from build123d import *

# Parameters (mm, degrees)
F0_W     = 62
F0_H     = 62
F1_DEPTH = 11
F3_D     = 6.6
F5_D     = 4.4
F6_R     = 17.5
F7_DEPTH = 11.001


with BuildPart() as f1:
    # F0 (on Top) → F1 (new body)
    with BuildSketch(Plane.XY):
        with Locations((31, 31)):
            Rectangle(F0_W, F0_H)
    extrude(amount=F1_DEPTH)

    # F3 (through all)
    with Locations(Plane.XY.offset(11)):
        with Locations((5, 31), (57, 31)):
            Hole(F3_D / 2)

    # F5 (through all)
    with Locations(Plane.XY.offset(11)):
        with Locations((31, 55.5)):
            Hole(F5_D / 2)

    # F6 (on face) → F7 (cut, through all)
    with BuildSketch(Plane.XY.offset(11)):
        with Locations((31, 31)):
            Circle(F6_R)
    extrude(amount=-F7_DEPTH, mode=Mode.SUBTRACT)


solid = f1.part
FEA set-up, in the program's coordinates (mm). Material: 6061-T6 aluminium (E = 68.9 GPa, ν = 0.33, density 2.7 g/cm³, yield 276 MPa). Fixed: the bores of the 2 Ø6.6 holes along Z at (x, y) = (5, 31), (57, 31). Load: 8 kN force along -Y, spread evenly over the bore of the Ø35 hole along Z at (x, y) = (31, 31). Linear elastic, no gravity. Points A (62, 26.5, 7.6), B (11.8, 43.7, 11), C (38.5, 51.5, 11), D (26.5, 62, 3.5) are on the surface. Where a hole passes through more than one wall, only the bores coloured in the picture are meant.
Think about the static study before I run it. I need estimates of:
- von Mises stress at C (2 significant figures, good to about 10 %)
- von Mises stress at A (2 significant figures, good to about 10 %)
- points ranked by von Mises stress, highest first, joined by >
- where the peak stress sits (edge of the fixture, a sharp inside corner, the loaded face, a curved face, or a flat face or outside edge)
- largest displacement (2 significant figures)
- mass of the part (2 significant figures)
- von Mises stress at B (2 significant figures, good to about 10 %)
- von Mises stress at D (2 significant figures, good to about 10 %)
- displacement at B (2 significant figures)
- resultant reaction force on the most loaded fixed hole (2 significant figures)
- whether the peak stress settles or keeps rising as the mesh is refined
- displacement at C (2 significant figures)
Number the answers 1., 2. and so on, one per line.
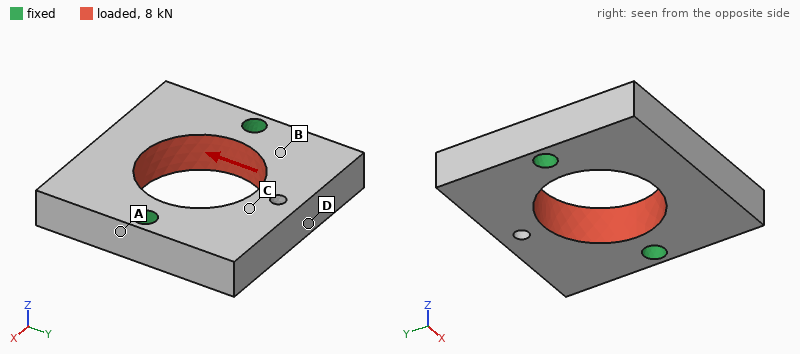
1. 8.7 MPa
2. 3.5 MPa
3. D > B > C > A
4. edge of the fixture
5. 9.3 µm
6. 83 g
7. 12 MPa
8. 18 MPa
9. 3.1 µm
10. 4.0 kN
11. keeps rising
12. 7.4 µm
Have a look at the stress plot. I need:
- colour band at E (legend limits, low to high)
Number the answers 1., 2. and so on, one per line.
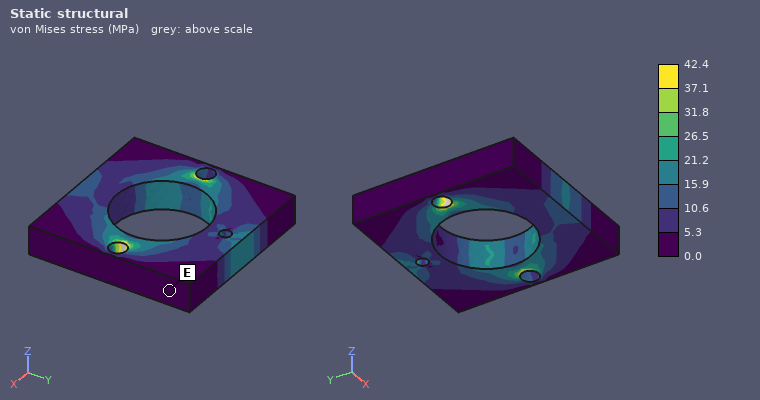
1. 0.0 to 5.3 MPa
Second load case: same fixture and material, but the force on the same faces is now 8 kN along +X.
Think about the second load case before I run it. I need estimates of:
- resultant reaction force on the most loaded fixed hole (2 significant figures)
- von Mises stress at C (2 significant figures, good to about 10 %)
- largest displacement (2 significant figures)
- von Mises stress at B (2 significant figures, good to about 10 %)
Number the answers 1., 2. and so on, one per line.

1. 4.0 kN
2. 6.1 MPa
3. 12 µm
4. 14 MPa
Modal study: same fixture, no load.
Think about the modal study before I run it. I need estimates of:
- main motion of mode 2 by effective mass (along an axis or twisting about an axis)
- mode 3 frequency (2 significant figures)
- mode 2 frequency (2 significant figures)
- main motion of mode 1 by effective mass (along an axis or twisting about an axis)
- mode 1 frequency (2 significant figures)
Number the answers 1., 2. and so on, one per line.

1. along Z
2. 11 kHz
3. 6500 Hz
4. twisting about X
5. 6200 Hz
